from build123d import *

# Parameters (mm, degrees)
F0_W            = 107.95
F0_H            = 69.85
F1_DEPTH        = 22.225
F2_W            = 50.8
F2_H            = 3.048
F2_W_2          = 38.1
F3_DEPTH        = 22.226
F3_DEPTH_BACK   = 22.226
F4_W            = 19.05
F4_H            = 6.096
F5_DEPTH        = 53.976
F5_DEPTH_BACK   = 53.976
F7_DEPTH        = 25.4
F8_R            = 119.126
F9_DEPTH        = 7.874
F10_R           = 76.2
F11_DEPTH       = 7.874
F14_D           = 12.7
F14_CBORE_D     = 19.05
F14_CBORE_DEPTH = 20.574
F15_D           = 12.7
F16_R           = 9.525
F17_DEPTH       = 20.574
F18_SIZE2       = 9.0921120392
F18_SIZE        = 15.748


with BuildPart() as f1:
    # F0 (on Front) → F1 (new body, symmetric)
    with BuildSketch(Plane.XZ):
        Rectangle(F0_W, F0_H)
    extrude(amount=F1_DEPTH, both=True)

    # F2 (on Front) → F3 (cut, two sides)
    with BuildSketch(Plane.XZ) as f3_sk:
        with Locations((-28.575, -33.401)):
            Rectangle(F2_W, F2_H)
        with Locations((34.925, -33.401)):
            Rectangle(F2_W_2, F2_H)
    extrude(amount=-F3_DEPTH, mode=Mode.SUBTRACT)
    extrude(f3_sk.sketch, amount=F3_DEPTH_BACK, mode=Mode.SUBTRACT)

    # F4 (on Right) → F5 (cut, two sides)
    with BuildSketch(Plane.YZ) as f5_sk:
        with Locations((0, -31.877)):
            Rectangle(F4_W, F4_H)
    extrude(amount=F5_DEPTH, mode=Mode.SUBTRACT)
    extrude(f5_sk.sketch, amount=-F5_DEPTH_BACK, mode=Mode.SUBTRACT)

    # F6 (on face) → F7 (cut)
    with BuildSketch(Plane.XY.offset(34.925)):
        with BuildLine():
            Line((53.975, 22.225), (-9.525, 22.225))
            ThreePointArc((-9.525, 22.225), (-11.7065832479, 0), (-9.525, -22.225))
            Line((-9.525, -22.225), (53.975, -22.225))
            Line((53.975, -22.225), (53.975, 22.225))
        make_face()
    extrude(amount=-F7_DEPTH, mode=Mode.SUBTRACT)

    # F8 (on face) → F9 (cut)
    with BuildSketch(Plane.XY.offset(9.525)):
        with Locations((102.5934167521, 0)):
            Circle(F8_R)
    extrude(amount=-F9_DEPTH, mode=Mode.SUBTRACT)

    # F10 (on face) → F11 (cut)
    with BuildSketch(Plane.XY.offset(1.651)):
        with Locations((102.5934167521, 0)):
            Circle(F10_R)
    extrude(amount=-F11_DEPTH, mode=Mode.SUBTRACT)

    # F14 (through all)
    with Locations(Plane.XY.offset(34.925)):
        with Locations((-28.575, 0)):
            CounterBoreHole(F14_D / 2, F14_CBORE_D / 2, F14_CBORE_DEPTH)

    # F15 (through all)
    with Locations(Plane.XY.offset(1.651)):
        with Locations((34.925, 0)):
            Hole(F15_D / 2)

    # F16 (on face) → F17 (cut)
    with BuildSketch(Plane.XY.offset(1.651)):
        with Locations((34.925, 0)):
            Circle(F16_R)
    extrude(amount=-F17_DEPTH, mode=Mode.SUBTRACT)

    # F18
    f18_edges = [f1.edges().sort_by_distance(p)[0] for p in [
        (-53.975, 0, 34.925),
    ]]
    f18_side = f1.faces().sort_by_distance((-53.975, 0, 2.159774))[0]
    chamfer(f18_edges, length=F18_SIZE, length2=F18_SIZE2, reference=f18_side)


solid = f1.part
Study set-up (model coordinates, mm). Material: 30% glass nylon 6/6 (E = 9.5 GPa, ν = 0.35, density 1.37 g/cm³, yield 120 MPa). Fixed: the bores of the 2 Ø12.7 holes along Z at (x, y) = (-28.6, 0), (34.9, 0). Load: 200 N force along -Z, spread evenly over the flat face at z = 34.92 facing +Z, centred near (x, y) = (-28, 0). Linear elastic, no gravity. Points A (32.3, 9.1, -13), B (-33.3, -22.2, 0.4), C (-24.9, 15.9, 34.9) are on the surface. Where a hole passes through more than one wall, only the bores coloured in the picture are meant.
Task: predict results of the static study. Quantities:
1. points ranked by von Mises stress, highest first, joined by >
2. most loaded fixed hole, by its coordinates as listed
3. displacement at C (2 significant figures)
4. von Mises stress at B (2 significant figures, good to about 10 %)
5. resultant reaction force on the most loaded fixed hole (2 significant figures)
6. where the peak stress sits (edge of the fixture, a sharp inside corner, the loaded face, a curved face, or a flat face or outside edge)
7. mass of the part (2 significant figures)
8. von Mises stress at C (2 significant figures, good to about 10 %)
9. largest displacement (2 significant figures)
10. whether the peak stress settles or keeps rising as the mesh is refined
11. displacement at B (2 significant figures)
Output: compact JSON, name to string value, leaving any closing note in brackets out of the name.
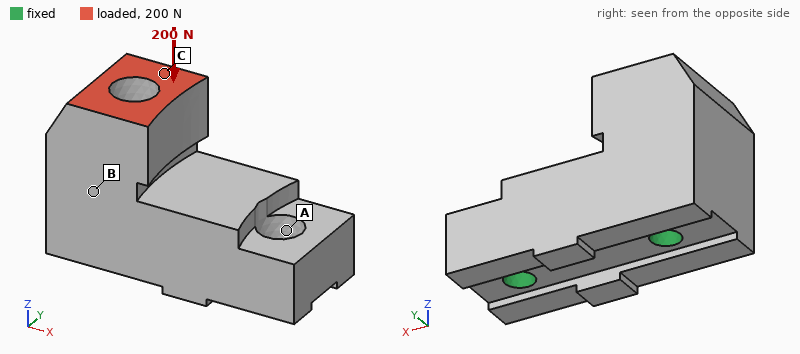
{"points ranked by von Mises stress, highest first, joined by >": "C > B > A", "most loaded fixed hole, by its coordinates as listed": "(-28.6, 0)", "displacement at C": "0.92 µm", "von Mises stress at B": "0.078 MPa", "resultant reaction force on the most loaded fixed hole": "200 N", "where the peak stress sits": "edge of the fixture", "mass of the part": "260 g", "von Mises stress at C": "0.17 MPa", "largest displacement": "1.2 µm", "whether the peak stress settles or keeps rising as the mesh is refined": "keeps rising", "displacement at B": "0.27 µm"}
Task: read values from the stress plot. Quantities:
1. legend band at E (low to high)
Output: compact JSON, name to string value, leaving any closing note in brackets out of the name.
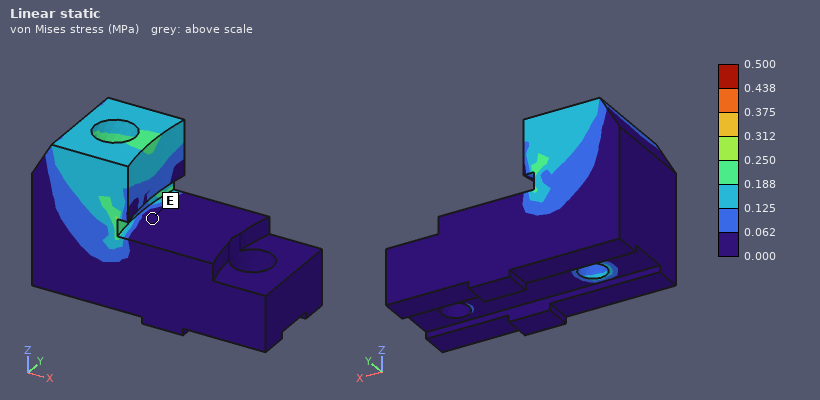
{"legend band at E": "0.000 to 0.062 MPa"}
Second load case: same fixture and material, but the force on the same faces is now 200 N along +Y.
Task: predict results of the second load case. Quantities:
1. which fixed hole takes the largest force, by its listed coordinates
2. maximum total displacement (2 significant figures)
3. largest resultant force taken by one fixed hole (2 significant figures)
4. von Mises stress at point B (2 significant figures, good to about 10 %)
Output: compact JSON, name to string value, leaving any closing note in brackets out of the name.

{"which fixed hole takes the largest force, by its listed coordinates": "(-28.6, 0)", "maximum total displacement": "5.1 µm", "largest resultant force taken by one fixed hole": "200 N", "von Mises stress at point B": "0.32 MPa"}
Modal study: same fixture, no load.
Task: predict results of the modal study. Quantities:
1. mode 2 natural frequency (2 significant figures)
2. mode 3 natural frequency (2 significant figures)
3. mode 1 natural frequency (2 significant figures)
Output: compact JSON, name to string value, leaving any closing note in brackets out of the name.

{"mode 2 natural frequency": "6900 Hz", "mode 3 natural frequency": "7000 Hz", "mode 1 natural frequency": "5800 Hz"}
